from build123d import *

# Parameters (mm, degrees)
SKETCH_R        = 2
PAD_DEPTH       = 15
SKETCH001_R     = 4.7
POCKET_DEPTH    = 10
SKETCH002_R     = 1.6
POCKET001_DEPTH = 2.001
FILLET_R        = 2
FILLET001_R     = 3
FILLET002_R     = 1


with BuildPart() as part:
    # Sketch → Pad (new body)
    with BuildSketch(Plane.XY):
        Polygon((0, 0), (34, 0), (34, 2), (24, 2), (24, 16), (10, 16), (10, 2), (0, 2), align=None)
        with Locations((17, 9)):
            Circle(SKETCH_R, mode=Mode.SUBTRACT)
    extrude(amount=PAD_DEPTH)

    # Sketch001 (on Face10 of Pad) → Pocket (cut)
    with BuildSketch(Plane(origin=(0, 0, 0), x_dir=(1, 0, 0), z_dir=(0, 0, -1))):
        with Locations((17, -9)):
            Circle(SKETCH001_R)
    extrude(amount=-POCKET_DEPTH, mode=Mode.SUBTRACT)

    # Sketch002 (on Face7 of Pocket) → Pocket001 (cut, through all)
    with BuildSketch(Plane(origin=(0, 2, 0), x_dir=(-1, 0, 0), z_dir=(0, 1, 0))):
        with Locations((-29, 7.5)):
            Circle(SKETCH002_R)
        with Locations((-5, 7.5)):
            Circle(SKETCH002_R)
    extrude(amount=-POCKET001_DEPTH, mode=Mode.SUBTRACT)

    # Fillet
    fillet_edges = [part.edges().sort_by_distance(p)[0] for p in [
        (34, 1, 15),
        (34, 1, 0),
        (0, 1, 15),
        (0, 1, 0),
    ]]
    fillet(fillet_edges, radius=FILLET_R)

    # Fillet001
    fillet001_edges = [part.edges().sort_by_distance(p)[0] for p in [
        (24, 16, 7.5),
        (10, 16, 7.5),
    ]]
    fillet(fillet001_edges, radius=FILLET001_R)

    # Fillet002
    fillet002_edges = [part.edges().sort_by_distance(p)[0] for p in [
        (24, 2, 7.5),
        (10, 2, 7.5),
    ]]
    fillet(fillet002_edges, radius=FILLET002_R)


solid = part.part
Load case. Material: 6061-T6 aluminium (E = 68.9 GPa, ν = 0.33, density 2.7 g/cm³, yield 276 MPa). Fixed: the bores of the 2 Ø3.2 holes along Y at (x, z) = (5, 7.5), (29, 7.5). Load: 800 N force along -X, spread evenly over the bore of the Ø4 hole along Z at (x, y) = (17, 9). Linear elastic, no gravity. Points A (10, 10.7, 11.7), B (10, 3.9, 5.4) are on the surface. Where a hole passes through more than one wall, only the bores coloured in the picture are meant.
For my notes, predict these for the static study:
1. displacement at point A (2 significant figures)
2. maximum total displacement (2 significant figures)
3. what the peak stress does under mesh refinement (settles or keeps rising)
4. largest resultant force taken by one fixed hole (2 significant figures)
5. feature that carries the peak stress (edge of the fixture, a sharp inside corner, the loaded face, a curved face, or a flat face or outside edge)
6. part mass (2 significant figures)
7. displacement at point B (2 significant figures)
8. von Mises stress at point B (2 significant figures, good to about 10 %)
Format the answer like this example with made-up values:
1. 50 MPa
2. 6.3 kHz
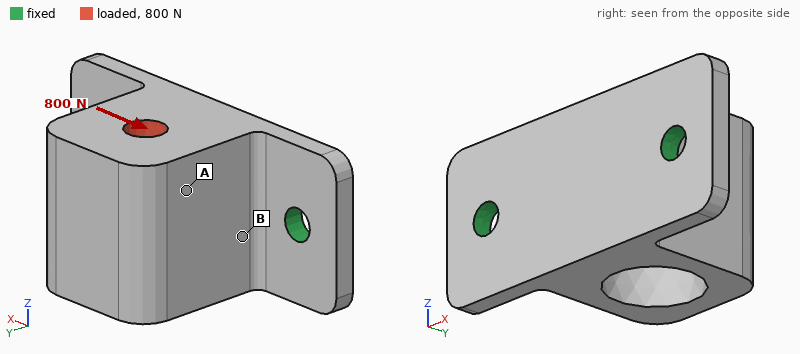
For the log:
1. 18 µm
2. 24 µm
3. keeps rising
4. 550 N
5. edge of the fixture
6. 8.4 g
7. 8.2 µm
8. 23 MPa
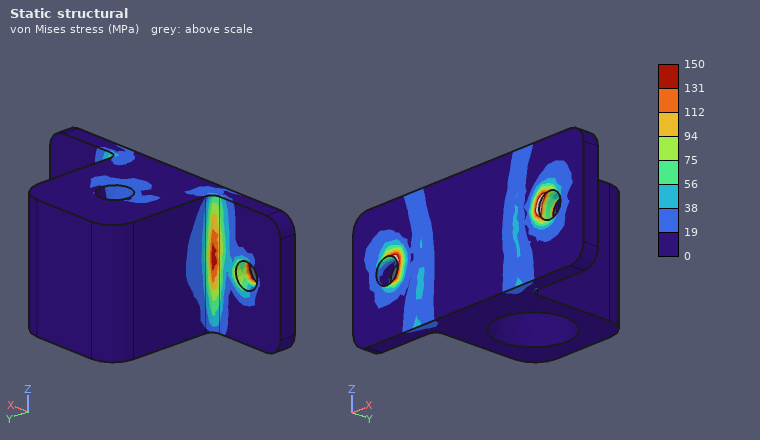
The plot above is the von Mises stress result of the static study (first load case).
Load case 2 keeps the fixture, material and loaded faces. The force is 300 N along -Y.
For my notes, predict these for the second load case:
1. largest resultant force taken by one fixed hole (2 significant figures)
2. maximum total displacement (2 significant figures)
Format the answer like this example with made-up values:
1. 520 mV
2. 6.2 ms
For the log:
1. 170 N
2. 42 µm
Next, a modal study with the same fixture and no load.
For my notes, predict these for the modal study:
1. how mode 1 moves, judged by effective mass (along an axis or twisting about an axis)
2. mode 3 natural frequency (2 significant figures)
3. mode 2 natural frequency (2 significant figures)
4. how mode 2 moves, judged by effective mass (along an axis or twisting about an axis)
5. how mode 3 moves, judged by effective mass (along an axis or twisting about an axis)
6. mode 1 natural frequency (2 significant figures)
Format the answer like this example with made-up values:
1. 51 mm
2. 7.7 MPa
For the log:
1. along Z
2. 15 kHz
3. 14 kHz
4. along X
5. along Y
6. 5000 Hz
